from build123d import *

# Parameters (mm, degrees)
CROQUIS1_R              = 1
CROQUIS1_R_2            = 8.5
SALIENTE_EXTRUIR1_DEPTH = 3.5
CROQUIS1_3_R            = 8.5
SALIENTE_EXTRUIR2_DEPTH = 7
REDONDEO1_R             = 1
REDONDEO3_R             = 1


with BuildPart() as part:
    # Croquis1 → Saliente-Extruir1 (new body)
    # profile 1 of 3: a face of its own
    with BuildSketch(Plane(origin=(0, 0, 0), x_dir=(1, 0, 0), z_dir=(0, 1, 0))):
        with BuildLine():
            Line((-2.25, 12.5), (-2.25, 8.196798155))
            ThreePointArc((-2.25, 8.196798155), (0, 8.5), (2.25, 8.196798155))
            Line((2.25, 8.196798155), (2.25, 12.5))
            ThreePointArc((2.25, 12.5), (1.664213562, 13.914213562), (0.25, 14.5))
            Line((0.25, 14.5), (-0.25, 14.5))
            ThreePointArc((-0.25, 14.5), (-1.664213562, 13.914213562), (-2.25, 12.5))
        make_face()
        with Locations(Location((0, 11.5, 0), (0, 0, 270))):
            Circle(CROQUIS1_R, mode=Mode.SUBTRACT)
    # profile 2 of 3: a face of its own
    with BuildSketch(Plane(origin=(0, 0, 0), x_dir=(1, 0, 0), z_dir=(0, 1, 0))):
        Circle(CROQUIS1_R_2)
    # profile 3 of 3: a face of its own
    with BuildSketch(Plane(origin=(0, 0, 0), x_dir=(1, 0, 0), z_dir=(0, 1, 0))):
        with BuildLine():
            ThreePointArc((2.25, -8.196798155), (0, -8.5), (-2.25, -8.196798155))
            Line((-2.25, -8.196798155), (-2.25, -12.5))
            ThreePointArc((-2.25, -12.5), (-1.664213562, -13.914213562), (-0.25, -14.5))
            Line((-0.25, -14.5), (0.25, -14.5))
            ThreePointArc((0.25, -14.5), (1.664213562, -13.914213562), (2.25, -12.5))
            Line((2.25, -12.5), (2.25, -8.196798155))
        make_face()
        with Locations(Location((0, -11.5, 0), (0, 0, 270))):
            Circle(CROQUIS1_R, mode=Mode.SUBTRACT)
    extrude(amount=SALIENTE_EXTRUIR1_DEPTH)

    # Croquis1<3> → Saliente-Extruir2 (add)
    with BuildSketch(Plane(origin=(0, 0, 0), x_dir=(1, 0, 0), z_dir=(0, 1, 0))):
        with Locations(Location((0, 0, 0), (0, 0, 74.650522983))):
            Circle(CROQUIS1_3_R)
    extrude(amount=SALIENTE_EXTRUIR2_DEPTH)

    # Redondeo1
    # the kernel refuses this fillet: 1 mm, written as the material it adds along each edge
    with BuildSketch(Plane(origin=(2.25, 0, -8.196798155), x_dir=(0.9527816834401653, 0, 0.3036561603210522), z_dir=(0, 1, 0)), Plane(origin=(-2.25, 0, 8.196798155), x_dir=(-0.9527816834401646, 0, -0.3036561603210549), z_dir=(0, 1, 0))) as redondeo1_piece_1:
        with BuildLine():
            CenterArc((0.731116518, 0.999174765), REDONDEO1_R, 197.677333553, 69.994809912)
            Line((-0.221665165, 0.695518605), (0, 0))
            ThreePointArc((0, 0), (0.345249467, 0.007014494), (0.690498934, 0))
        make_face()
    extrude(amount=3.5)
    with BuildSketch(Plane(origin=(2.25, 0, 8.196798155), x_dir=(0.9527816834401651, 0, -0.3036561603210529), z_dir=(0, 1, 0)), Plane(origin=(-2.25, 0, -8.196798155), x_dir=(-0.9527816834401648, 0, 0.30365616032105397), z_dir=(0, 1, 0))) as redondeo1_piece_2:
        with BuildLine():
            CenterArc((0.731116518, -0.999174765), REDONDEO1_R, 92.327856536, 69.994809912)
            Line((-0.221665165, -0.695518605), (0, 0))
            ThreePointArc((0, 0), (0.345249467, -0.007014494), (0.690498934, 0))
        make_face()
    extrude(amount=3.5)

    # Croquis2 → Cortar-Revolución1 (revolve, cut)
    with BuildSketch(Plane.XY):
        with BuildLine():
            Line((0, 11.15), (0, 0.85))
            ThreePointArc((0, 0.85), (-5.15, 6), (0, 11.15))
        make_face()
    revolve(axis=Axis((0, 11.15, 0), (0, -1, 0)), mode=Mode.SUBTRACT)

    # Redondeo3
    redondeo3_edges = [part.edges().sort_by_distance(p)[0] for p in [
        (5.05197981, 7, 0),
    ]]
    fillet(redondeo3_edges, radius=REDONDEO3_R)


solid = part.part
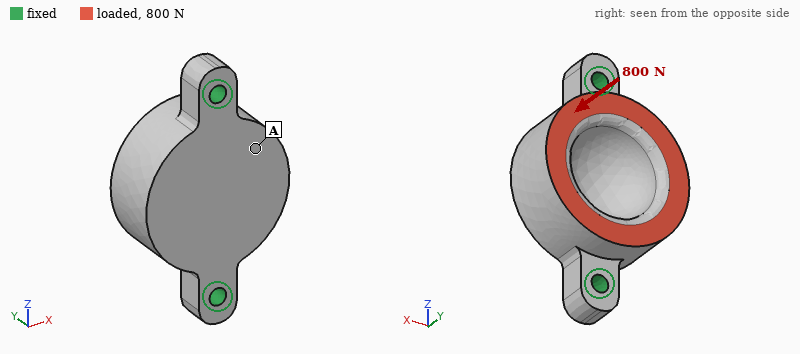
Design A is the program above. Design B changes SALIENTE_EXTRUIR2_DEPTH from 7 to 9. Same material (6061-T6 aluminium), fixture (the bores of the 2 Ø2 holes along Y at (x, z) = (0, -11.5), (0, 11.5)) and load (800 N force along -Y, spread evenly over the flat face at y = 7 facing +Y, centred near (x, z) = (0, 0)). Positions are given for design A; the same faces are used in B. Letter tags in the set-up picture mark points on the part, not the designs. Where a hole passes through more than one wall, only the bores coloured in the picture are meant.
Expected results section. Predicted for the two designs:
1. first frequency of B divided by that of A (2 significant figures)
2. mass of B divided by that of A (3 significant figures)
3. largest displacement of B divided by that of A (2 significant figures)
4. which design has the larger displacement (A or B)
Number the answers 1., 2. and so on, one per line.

1. 0.80
2. 1.22
3. 0.74
4. A
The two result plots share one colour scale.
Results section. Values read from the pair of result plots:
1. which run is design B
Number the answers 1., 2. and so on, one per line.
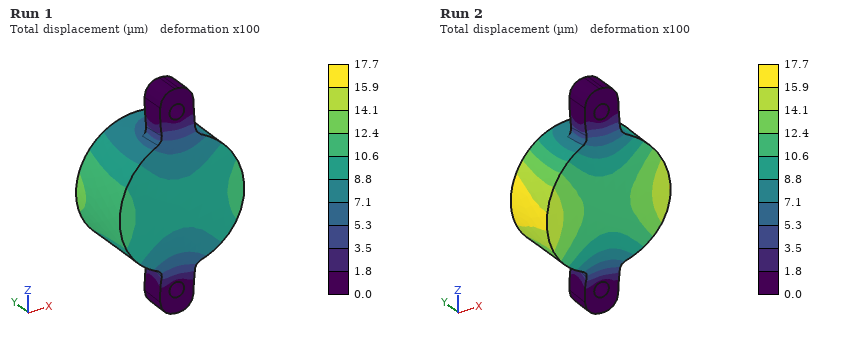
1. Run 1
